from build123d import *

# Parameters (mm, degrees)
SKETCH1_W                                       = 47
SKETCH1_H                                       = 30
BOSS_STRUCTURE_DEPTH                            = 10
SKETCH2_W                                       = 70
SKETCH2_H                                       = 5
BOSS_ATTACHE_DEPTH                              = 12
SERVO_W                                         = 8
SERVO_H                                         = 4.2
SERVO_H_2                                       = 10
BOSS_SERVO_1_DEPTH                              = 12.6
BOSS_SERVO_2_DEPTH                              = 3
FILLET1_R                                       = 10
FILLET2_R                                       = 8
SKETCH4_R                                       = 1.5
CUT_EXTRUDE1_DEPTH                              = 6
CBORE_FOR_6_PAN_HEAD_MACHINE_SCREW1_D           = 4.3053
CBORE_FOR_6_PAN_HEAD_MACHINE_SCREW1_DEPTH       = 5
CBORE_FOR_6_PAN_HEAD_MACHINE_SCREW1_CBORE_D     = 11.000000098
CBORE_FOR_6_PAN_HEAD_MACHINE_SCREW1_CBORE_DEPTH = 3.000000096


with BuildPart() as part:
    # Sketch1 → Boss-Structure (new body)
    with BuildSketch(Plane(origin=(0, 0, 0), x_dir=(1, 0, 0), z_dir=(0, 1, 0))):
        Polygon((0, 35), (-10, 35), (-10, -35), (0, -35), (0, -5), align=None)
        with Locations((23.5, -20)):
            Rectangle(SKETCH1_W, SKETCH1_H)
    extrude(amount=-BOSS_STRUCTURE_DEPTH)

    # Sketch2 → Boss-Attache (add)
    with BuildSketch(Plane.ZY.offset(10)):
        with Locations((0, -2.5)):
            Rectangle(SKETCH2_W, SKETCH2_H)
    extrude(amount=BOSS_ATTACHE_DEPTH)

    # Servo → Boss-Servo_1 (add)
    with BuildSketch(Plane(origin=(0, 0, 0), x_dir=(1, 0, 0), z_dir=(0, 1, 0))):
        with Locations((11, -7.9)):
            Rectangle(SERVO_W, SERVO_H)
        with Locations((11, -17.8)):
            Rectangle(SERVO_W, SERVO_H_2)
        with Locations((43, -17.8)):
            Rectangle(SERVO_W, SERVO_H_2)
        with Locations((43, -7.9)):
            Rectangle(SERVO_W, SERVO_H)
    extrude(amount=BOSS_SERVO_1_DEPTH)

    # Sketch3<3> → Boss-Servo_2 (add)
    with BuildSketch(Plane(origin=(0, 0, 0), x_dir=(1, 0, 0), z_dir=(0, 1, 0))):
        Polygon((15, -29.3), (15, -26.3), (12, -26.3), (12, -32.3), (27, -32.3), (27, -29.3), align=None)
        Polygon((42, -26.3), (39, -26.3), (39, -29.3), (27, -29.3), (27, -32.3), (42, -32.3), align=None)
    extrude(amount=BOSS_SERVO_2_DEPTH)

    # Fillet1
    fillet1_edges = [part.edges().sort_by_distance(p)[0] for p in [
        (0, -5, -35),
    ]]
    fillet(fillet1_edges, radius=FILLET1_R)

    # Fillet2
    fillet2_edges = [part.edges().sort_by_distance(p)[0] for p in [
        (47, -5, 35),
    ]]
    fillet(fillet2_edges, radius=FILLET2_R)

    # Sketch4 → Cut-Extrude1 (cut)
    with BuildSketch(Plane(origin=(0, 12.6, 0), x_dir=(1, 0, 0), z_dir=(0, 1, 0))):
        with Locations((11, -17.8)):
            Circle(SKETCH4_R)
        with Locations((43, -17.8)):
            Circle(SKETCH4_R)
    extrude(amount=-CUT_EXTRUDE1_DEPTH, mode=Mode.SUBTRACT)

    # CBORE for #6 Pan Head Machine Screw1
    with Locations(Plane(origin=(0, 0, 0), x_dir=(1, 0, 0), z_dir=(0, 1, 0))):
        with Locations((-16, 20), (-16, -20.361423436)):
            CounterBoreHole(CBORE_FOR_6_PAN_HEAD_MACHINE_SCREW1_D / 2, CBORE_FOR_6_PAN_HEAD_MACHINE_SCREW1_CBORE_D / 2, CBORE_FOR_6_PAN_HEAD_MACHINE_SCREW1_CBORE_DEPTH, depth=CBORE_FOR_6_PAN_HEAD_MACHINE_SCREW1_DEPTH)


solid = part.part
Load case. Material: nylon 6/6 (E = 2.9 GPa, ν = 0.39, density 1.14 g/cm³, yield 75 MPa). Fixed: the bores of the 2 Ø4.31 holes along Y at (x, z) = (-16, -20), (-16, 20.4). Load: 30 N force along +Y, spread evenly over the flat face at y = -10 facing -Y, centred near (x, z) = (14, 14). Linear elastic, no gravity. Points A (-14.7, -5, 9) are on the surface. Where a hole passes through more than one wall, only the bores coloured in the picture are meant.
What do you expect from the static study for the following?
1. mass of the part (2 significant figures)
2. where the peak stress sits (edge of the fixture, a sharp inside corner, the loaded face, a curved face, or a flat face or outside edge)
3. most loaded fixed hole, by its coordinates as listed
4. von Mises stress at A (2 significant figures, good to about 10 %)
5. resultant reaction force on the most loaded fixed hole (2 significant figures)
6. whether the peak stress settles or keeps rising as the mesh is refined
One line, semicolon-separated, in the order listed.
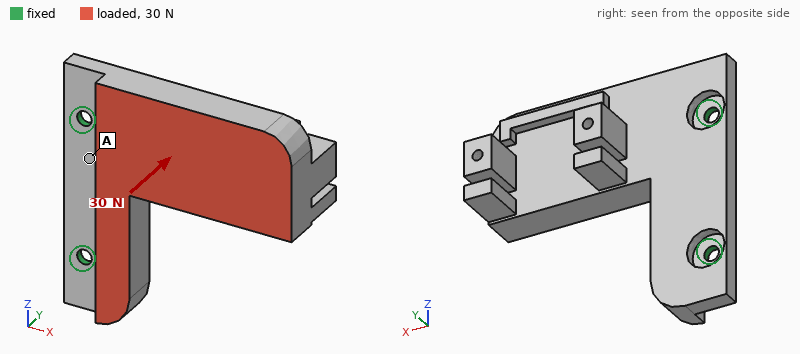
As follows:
31 g; edge of the fixture; (-16, 20.4); 2.3 MPa; 25 N; keeps rising
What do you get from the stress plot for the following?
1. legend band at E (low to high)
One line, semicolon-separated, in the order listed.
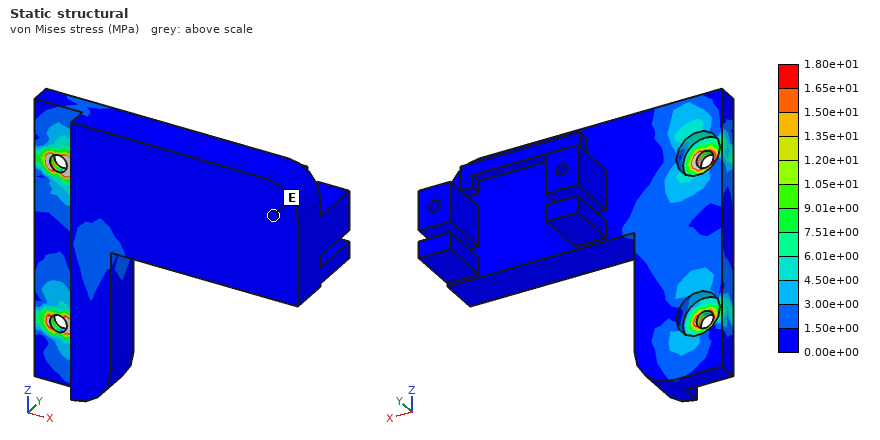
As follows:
0.00e+00 to 1.50e+00 MPa
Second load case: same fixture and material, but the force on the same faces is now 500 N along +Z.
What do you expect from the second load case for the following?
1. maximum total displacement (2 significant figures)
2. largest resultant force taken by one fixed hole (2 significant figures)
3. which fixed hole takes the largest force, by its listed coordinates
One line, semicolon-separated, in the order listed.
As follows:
0.69 mm; 530 N; (-16, -20)
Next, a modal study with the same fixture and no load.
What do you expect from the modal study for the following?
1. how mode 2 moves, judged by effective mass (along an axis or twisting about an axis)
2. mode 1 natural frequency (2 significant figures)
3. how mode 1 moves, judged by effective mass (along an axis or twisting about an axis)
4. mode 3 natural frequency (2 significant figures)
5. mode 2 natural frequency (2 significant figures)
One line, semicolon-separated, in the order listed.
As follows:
along Z; 190 Hz; along Y; 1400 Hz; 990 Hz
